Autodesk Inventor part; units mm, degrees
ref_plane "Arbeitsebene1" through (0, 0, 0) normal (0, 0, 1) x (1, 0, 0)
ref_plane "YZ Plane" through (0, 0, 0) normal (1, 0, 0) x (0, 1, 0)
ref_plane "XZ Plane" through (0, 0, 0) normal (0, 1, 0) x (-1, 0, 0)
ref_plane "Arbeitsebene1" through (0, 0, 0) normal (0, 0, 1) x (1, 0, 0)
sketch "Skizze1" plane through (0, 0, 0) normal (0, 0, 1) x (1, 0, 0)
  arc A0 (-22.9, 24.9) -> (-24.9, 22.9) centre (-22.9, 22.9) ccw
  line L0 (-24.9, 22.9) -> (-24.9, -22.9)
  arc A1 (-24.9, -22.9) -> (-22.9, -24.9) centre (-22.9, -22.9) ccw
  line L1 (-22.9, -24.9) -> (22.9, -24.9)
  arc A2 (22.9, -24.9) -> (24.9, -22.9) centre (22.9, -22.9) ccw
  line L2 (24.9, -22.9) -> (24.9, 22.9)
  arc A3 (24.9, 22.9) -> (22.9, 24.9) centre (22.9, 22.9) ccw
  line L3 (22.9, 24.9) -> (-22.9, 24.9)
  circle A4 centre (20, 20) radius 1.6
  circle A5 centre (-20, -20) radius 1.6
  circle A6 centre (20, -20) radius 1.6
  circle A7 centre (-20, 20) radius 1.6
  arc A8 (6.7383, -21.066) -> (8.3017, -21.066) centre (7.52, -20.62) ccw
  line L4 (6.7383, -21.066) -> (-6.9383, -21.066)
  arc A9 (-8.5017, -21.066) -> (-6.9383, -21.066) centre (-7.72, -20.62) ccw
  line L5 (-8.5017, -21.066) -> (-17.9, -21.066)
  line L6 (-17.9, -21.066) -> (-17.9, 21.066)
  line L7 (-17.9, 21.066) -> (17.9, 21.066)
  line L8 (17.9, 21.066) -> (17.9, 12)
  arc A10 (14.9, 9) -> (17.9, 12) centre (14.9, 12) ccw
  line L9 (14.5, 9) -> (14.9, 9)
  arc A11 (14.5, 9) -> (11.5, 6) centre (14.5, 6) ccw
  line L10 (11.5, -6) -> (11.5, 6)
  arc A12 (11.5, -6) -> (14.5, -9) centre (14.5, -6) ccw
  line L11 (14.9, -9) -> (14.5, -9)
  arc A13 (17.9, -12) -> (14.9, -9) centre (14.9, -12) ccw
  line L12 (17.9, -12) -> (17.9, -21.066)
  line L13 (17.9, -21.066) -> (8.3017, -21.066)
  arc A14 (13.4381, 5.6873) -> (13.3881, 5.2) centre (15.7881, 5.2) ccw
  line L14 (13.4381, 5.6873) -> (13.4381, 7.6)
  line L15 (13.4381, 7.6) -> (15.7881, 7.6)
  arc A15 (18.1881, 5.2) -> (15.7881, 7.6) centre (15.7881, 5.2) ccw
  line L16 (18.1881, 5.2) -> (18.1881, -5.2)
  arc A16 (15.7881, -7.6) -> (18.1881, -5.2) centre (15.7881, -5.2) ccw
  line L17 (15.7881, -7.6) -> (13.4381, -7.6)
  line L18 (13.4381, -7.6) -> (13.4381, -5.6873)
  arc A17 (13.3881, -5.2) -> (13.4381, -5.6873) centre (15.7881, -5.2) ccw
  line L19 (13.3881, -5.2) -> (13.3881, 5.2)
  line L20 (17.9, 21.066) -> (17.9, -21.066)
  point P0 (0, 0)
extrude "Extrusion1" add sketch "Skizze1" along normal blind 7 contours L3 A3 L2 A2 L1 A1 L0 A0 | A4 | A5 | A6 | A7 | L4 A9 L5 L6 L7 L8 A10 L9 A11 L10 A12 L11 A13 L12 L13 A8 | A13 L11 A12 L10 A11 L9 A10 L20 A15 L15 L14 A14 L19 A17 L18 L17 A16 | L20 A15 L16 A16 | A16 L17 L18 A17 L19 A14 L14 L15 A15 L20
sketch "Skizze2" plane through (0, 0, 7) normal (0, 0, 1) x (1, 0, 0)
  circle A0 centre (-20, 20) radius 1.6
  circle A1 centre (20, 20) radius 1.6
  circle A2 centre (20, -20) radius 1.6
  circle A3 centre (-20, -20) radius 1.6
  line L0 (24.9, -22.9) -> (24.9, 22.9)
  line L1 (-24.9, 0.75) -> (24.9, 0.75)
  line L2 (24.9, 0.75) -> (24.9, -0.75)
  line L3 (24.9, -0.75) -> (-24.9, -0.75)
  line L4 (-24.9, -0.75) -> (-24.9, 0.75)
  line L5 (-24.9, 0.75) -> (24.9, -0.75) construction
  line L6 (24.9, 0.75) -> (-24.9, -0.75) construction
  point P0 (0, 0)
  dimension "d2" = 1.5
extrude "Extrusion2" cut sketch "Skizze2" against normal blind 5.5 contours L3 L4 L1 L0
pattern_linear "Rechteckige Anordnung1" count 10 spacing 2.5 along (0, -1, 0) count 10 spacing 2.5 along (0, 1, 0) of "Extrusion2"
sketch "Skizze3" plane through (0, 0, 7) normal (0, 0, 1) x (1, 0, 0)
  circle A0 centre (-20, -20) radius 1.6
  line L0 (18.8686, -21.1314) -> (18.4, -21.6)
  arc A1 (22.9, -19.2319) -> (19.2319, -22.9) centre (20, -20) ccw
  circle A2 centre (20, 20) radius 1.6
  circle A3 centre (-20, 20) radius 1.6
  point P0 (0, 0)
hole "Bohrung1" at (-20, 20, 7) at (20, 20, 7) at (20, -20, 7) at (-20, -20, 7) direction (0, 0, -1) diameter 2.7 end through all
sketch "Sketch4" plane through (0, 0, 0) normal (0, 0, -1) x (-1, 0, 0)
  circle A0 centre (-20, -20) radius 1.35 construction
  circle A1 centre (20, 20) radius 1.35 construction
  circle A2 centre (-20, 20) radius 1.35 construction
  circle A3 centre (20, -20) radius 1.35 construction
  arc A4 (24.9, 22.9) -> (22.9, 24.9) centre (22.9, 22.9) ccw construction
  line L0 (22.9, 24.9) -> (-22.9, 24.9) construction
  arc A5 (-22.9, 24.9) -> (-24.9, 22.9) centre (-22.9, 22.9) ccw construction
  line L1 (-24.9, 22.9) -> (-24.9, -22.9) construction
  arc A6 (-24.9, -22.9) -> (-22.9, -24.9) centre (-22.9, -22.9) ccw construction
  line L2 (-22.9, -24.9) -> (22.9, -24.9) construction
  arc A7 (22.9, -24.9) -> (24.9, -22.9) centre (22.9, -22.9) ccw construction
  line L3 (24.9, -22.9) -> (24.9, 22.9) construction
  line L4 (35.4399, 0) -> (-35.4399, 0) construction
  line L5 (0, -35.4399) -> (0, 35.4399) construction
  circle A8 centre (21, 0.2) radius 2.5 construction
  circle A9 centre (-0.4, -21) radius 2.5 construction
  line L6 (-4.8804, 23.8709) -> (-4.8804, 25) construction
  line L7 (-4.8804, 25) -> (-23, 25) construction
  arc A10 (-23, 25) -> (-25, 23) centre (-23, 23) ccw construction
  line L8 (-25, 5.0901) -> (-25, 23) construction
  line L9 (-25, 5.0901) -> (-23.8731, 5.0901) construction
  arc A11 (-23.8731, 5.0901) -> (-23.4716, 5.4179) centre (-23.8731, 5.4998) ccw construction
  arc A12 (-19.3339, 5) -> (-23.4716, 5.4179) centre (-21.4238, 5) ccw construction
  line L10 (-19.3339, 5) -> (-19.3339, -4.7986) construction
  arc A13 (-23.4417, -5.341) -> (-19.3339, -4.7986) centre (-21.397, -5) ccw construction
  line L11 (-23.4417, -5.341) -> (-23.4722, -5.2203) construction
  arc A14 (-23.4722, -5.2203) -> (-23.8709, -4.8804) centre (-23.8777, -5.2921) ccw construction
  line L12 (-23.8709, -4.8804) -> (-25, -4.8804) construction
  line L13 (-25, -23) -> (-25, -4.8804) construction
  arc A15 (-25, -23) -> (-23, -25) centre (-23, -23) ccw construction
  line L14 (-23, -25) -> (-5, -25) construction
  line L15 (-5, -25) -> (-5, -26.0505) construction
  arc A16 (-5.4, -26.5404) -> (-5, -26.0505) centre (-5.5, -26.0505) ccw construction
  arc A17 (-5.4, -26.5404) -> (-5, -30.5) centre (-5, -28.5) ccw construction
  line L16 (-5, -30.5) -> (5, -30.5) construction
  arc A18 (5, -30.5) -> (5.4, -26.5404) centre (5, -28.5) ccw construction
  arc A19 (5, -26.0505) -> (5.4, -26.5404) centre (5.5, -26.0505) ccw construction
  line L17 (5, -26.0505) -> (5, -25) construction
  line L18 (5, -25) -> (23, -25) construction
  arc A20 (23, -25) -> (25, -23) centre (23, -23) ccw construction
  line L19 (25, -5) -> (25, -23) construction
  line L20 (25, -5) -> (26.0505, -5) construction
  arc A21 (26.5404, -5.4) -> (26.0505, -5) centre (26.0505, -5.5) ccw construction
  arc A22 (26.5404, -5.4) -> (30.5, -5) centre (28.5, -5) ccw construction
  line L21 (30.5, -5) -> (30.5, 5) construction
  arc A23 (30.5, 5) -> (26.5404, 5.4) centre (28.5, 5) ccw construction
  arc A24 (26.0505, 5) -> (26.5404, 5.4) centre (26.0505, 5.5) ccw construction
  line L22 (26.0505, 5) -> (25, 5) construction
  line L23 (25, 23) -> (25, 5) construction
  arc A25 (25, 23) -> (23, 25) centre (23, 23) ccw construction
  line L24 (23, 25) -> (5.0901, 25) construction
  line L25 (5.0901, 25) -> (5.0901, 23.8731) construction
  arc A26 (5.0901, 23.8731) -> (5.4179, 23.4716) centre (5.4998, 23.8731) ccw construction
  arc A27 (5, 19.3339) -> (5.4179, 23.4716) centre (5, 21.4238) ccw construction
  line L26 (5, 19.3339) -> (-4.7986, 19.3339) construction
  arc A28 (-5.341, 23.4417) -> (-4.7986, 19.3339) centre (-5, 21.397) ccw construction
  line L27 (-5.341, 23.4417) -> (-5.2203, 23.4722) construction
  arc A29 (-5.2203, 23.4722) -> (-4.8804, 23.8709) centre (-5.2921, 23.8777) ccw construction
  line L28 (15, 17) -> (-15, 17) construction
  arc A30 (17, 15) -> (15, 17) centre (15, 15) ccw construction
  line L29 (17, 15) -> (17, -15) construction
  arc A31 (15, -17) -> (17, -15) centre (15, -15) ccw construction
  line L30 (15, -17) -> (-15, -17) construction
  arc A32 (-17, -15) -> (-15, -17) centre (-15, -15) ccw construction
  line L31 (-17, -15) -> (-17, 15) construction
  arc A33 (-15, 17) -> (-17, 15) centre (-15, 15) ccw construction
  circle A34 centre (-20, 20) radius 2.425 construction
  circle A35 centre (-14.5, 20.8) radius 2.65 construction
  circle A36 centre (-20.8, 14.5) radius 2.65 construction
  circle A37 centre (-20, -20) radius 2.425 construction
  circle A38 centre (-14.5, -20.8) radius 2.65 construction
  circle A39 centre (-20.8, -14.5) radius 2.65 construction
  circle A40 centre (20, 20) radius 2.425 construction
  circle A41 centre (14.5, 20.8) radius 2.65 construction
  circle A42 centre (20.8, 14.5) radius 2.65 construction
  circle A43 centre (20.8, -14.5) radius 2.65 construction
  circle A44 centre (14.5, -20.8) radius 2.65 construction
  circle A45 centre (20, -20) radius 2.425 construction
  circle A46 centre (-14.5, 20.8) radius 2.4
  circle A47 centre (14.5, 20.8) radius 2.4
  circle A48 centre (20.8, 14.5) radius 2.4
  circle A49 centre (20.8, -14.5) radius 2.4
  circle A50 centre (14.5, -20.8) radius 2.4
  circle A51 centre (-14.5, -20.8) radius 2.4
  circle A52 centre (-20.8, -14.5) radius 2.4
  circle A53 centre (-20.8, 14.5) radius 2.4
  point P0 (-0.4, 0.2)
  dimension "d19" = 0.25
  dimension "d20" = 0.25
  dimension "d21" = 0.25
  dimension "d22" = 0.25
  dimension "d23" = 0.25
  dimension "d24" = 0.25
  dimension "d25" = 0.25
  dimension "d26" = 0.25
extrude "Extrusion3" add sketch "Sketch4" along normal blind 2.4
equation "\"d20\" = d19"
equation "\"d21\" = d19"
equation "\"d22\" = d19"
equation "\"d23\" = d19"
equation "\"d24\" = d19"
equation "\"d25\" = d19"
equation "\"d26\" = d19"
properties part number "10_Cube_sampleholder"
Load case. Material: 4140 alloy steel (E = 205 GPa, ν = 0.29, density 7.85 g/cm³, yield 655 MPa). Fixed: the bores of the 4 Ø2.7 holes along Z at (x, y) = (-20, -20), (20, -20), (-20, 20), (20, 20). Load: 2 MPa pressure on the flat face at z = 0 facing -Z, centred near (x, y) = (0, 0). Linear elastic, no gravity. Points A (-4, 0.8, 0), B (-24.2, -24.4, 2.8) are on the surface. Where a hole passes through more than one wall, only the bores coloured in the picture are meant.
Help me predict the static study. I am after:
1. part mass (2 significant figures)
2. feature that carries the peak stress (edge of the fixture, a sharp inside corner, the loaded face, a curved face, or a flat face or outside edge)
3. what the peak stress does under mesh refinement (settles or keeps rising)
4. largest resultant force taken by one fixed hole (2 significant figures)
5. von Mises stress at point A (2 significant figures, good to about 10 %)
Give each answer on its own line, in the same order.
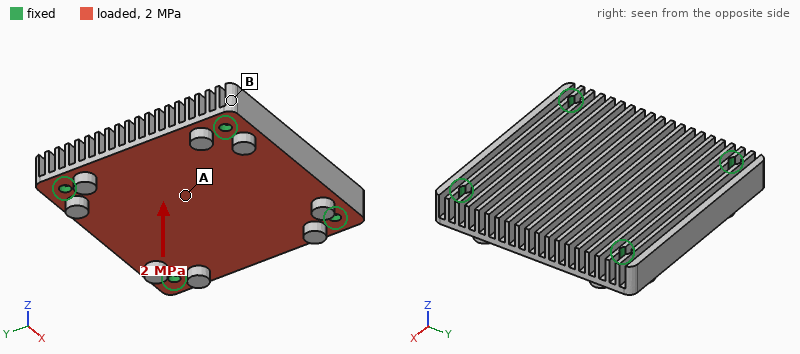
77 g
edge of the fixture
keeps rising
1.2 kN
260 MPa
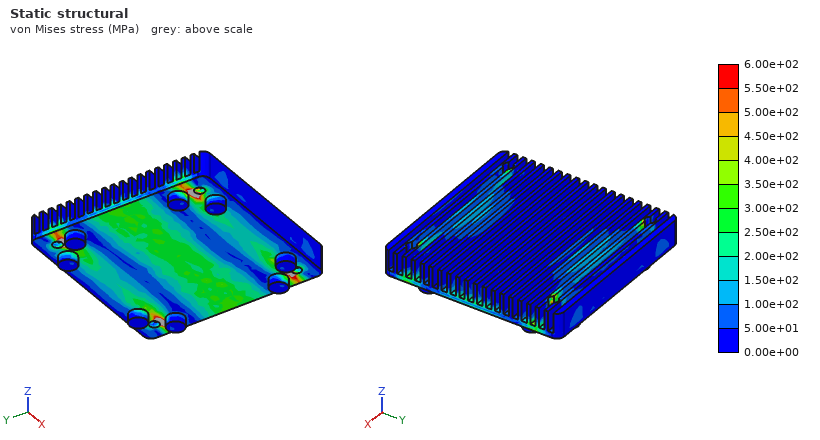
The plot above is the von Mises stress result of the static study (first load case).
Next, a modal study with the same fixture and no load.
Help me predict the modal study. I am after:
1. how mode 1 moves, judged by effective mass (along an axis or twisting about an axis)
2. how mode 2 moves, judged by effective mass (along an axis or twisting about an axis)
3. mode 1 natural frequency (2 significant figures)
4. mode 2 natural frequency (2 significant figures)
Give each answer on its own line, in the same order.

along Z
twisting about Y
3200 Hz
4200 Hz
